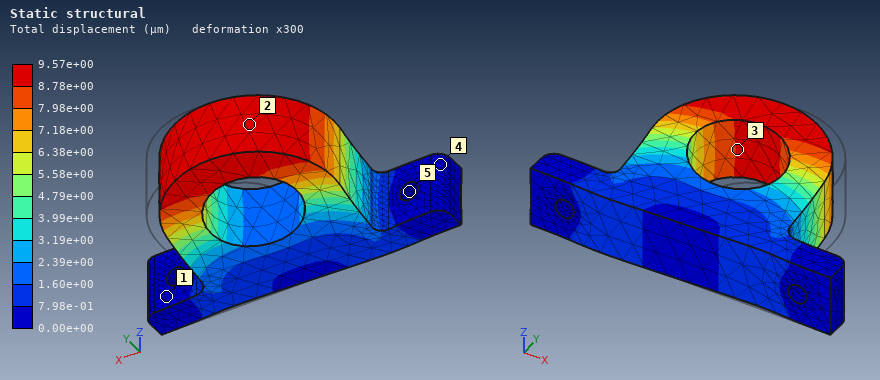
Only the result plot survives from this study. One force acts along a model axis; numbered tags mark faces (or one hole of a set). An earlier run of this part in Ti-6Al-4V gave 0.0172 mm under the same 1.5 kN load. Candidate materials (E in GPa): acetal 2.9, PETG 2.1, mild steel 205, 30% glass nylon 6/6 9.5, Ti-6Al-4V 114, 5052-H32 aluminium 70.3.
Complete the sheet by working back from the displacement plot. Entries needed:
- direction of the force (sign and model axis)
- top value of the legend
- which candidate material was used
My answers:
-X
9.57e+00 µm
mild steel
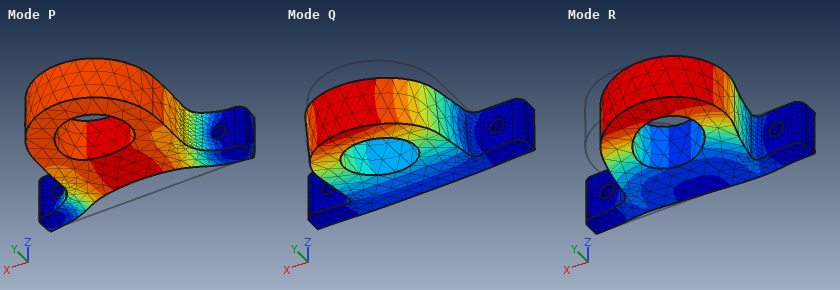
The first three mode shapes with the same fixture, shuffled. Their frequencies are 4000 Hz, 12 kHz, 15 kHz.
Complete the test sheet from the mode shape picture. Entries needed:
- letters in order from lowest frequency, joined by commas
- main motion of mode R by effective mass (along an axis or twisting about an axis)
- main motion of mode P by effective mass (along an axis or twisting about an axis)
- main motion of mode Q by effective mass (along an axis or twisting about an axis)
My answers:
Q, R, P
along X
along Y
along Z
